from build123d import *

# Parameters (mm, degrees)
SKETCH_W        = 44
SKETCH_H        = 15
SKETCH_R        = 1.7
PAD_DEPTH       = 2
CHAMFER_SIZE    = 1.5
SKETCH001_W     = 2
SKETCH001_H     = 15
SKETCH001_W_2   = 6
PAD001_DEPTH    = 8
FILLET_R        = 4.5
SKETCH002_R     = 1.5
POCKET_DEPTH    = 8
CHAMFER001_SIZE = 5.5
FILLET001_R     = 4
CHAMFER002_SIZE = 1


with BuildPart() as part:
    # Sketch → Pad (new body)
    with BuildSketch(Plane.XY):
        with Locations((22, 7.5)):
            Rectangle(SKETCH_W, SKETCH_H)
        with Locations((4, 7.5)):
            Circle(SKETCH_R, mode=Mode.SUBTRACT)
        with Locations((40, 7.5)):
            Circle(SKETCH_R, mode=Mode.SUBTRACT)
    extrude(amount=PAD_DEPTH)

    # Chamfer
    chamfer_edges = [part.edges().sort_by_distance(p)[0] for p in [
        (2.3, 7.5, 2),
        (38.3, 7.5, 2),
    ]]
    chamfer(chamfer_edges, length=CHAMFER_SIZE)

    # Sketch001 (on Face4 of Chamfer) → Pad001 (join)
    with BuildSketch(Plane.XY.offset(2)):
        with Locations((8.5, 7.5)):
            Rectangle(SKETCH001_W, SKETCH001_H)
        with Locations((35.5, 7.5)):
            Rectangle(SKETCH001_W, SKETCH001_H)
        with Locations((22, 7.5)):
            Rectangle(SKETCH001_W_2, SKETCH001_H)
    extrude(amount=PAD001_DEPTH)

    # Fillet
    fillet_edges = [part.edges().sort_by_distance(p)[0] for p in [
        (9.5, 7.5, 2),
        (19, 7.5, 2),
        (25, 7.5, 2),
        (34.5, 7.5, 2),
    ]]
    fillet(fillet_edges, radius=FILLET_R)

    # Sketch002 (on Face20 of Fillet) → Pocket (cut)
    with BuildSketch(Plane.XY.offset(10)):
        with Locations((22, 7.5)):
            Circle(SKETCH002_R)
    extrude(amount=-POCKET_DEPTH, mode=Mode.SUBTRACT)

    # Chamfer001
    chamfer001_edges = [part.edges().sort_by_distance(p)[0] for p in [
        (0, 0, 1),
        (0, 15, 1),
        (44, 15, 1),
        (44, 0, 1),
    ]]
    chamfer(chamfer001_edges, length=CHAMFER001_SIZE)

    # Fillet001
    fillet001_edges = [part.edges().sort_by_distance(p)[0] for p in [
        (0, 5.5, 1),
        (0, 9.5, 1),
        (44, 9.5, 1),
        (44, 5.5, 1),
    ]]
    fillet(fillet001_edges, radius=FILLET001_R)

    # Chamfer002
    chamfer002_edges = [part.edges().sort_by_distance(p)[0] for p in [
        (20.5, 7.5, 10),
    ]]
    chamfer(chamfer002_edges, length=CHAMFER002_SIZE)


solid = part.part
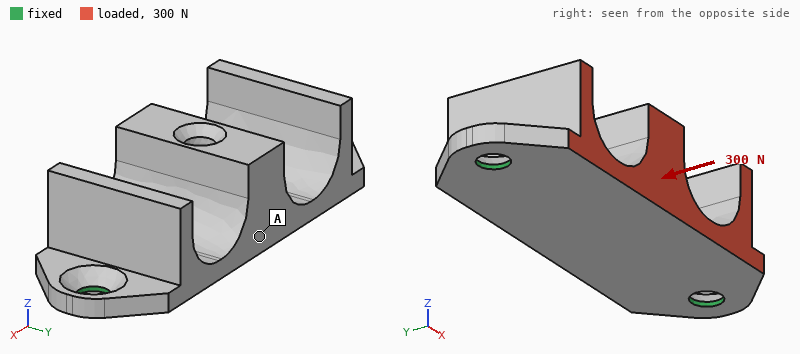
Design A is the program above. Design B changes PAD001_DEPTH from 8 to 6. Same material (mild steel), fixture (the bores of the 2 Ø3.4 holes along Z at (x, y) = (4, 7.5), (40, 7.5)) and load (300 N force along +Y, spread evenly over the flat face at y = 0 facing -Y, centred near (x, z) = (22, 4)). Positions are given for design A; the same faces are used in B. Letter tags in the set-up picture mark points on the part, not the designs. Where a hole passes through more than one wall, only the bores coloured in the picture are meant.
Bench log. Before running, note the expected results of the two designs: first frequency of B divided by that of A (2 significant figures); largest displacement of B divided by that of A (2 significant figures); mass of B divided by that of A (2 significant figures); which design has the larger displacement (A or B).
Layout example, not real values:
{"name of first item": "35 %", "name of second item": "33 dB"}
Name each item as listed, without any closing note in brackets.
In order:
{"first frequency of B divided by that of A": "1.2", "largest displacement of B divided by that of A": "0.69", "mass of B divided by that of A": "0.89", "which design has the larger displacement": "A"}
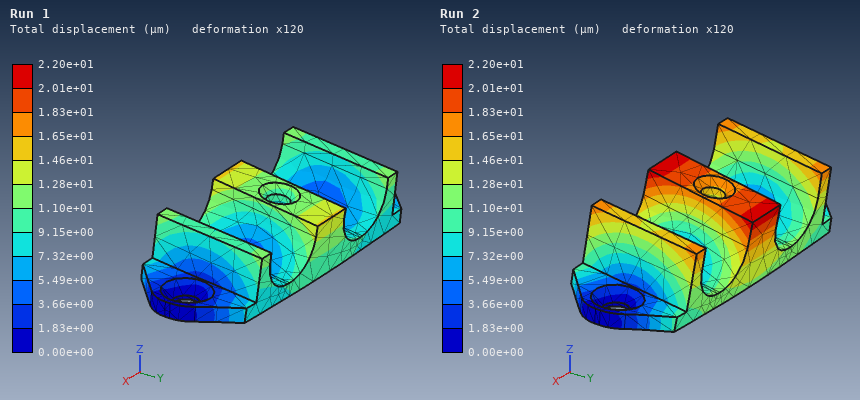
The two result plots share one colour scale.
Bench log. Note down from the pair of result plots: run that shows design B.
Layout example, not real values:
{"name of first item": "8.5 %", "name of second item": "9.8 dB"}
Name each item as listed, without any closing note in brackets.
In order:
{"run that shows design B": "Run 1"}
